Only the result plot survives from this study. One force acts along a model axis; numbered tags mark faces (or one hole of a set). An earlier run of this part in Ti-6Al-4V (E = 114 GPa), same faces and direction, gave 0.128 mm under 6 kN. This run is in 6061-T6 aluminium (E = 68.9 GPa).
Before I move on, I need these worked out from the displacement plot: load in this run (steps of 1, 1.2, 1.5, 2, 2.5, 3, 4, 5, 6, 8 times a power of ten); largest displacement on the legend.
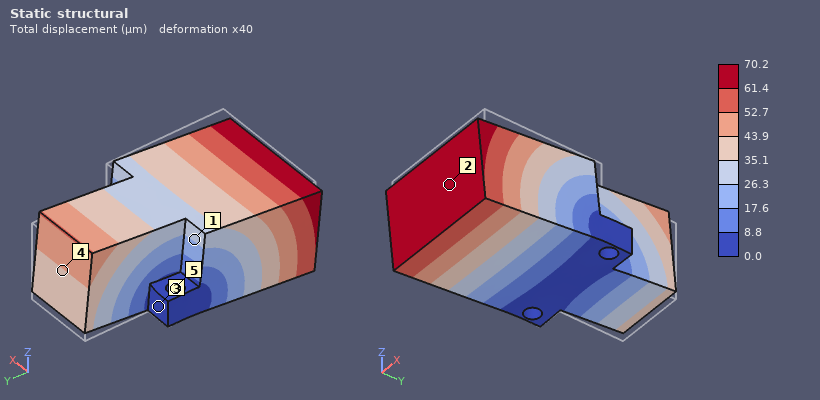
2 kN
70.2 µm
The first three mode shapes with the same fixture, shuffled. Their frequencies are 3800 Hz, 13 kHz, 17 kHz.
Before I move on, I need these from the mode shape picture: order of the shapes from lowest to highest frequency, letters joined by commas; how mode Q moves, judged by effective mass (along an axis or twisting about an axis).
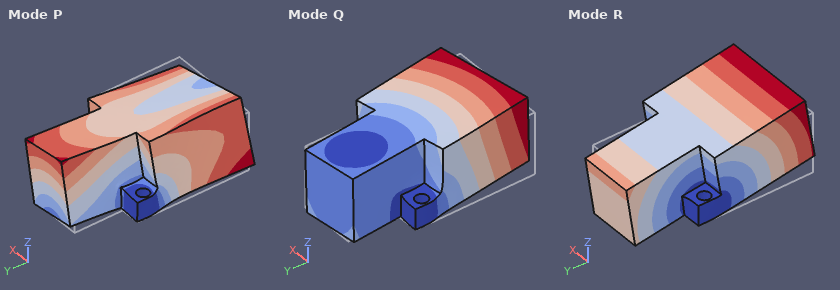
R, Q, P
along X
